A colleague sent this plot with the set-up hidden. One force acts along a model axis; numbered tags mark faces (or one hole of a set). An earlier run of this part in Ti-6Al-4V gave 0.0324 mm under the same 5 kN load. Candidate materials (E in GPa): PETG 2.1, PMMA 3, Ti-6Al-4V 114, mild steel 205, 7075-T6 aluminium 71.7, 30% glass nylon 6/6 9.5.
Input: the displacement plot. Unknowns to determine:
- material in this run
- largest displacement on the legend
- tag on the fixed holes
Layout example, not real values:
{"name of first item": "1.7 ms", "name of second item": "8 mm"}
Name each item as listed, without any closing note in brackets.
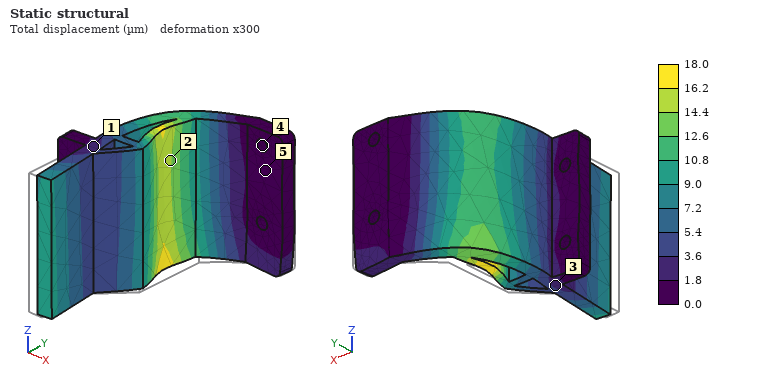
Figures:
{"material in this run": "mild steel", "largest displacement on the legend": "18.0 µm", "tag on the fixed holes": "4"}
